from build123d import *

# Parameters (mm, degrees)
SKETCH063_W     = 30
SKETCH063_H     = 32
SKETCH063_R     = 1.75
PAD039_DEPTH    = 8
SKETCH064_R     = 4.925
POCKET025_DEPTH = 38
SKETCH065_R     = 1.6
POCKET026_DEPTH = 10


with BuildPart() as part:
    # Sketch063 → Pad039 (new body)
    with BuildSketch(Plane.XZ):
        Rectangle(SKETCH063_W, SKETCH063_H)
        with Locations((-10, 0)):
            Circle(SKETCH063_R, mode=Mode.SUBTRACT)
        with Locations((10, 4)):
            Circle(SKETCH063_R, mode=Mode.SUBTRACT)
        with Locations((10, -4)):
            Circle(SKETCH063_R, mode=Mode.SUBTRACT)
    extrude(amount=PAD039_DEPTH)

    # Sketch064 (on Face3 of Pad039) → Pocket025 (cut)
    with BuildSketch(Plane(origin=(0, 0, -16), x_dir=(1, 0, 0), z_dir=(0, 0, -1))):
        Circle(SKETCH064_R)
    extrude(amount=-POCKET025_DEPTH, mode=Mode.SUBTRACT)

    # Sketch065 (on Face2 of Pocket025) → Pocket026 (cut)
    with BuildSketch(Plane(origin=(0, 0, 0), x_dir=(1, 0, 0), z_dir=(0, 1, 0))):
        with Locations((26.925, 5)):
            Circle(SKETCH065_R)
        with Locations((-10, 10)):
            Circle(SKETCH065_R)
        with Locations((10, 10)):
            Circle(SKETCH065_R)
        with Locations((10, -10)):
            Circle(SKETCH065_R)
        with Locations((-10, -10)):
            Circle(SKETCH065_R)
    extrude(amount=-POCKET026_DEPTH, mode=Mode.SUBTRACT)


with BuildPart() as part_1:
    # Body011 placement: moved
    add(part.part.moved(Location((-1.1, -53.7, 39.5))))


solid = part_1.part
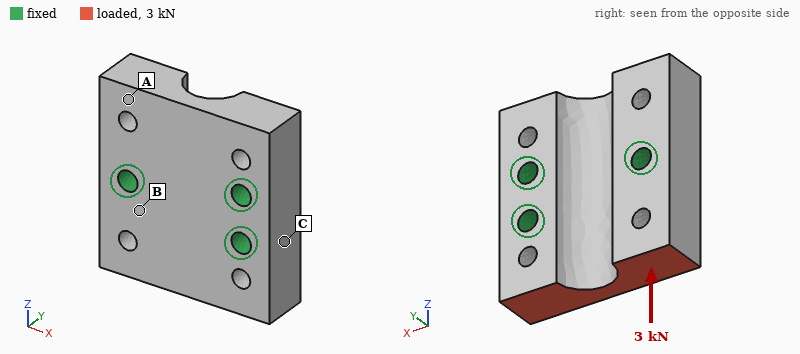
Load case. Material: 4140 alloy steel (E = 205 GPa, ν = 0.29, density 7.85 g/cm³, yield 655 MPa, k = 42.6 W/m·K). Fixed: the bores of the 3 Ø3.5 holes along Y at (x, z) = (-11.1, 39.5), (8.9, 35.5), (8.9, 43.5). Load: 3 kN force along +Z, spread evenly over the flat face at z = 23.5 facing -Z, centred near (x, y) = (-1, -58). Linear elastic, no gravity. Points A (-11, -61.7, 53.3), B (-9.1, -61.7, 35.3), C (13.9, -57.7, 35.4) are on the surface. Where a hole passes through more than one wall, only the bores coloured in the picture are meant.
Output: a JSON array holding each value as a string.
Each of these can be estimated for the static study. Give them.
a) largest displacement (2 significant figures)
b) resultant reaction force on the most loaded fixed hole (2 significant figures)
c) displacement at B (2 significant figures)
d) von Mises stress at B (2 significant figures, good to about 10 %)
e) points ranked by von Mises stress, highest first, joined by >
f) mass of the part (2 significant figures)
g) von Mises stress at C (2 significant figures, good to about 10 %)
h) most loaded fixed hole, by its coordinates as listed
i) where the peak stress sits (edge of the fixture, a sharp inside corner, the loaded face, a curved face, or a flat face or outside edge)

["1.6 µm", "1.5 kN", "0.40 µm", "21 MPa", "B > C > A", "47 g", "11 MPa", "(-11.1, 39.5)", "a curved face"]
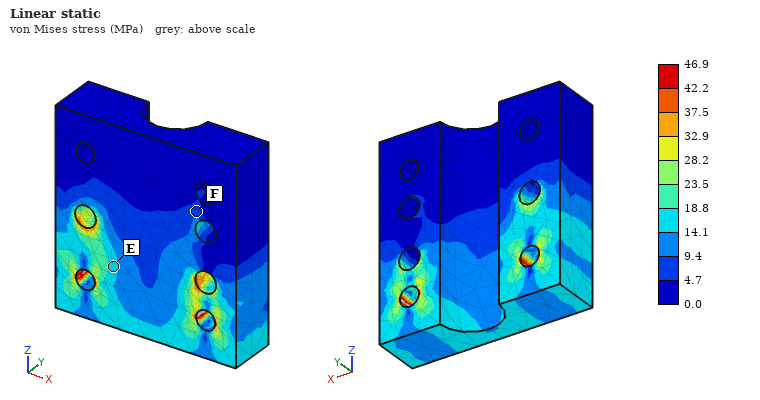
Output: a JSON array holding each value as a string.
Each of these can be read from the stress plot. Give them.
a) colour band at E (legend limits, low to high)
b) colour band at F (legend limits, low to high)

["14.1 to 18.8 MPa", "4.7 to 9.4 MPa"]
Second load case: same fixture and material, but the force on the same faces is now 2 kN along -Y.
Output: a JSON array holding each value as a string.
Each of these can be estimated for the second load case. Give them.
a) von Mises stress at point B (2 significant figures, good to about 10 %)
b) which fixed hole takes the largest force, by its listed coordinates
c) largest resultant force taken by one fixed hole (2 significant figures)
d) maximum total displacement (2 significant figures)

["76 MPa", "(8.9, 35.5)", "1.4 kN", "16 µm"]
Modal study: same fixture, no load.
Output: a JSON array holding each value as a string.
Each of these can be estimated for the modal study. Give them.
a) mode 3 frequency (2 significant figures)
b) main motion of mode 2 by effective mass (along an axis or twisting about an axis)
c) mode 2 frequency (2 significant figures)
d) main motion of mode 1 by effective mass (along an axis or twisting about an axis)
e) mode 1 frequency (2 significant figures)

["33 kHz", "along Y", "26 kHz", "twisting about X", "23 kHz"]
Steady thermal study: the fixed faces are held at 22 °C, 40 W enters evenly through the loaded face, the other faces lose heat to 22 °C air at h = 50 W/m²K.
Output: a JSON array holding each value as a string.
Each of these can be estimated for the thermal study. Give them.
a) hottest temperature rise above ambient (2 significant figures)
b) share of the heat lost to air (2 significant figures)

["75 K", "6.0 %"]
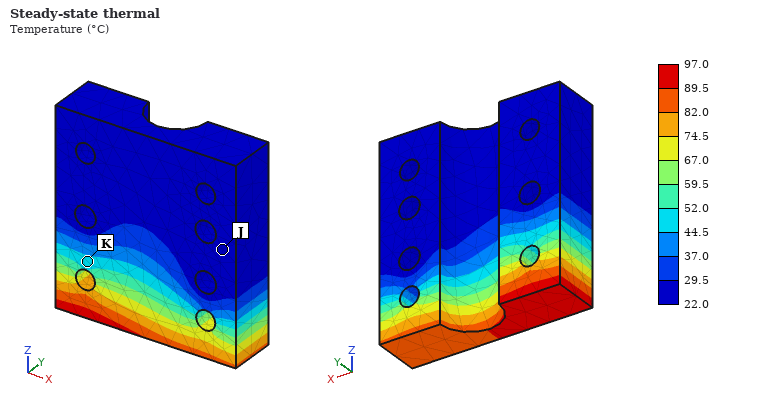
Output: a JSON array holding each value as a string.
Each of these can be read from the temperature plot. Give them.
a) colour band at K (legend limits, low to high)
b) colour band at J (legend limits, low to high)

["44.5 to 52.0 °C", "22.0 to 29.5 °C"]
